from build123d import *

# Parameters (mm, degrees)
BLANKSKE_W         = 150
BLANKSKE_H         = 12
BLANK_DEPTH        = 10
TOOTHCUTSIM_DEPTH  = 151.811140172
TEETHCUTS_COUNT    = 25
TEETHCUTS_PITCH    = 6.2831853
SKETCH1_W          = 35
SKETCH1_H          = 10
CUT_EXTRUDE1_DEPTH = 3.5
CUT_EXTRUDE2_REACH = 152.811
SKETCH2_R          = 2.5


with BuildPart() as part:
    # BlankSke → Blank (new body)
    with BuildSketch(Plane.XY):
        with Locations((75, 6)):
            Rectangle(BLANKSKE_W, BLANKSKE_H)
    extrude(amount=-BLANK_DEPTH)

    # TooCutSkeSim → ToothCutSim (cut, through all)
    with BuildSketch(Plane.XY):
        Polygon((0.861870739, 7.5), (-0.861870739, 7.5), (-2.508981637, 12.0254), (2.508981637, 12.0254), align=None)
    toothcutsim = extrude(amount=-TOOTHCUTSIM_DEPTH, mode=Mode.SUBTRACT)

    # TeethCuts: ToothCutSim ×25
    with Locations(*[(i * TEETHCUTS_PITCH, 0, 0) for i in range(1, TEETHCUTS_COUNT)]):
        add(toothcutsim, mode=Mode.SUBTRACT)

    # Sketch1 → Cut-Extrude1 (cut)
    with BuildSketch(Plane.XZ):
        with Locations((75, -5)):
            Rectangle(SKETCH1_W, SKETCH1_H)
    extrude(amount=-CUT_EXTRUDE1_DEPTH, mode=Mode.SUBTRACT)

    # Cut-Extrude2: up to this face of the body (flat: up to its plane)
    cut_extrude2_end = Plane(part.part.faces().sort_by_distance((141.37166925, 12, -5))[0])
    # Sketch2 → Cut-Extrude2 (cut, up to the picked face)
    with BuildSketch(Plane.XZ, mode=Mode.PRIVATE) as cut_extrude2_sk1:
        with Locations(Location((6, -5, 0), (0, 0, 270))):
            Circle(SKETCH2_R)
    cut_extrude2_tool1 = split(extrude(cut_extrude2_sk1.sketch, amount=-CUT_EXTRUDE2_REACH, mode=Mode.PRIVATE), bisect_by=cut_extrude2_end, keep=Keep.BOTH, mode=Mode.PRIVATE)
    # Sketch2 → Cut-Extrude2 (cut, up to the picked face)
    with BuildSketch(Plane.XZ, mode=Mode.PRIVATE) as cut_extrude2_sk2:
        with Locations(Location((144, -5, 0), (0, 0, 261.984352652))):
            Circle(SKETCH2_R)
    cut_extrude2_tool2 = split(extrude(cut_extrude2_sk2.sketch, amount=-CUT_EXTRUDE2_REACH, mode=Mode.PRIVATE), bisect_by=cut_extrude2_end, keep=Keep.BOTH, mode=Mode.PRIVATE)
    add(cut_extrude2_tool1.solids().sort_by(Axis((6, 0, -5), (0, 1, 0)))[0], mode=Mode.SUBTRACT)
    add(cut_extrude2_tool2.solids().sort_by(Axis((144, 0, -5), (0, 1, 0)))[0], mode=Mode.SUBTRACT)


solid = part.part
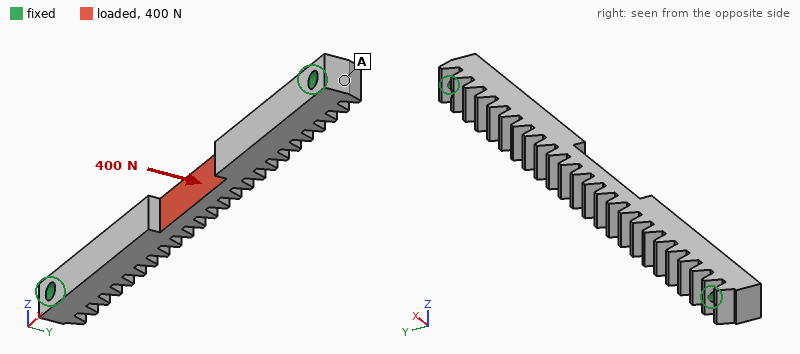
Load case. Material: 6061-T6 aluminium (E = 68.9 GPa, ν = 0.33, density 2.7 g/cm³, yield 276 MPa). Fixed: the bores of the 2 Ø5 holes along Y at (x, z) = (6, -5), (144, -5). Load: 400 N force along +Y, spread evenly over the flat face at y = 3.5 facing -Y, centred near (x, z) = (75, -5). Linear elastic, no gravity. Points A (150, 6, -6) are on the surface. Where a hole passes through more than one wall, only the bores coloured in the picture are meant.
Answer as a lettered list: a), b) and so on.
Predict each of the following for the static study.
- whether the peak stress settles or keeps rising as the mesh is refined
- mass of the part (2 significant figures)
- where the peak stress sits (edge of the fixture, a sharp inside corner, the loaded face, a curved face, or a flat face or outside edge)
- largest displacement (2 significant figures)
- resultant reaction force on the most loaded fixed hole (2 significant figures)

a) keeps rising
b) 35 g
c) edge of the fixture
d) 0.29 mm
e) 690 N
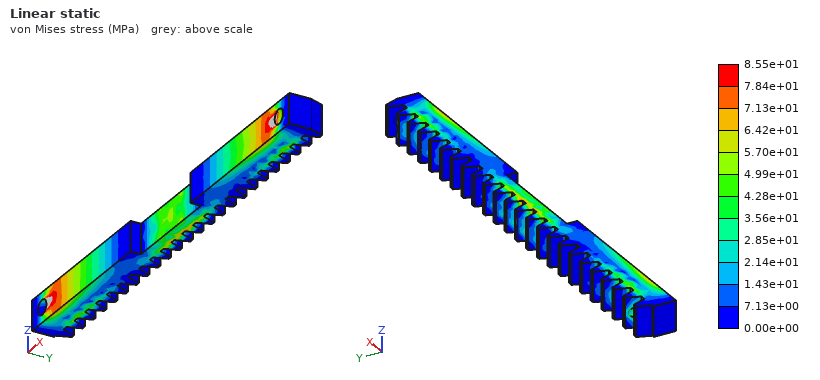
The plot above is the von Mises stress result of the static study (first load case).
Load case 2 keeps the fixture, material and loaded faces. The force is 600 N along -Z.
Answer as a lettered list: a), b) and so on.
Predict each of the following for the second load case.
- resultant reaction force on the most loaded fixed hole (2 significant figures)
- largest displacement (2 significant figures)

a) 300 N
b) 0.24 mm
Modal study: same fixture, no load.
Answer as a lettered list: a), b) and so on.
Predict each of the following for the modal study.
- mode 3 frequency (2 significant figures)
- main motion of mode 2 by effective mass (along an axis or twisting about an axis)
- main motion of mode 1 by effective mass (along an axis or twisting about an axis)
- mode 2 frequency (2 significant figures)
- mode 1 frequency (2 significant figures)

a) 4300 Hz
b) along Z
c) along Y
d) 2400 Hz
e) 1900 Hz
